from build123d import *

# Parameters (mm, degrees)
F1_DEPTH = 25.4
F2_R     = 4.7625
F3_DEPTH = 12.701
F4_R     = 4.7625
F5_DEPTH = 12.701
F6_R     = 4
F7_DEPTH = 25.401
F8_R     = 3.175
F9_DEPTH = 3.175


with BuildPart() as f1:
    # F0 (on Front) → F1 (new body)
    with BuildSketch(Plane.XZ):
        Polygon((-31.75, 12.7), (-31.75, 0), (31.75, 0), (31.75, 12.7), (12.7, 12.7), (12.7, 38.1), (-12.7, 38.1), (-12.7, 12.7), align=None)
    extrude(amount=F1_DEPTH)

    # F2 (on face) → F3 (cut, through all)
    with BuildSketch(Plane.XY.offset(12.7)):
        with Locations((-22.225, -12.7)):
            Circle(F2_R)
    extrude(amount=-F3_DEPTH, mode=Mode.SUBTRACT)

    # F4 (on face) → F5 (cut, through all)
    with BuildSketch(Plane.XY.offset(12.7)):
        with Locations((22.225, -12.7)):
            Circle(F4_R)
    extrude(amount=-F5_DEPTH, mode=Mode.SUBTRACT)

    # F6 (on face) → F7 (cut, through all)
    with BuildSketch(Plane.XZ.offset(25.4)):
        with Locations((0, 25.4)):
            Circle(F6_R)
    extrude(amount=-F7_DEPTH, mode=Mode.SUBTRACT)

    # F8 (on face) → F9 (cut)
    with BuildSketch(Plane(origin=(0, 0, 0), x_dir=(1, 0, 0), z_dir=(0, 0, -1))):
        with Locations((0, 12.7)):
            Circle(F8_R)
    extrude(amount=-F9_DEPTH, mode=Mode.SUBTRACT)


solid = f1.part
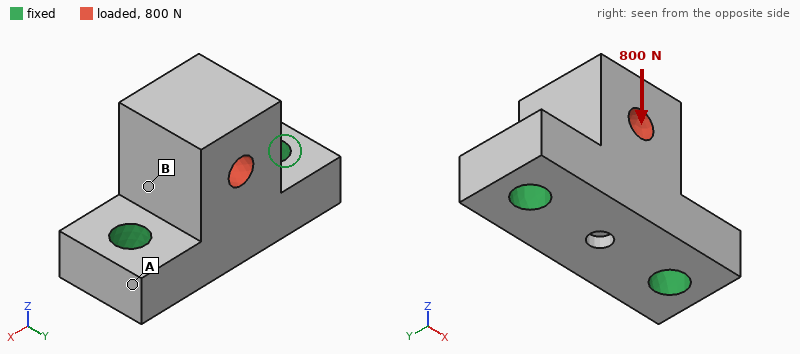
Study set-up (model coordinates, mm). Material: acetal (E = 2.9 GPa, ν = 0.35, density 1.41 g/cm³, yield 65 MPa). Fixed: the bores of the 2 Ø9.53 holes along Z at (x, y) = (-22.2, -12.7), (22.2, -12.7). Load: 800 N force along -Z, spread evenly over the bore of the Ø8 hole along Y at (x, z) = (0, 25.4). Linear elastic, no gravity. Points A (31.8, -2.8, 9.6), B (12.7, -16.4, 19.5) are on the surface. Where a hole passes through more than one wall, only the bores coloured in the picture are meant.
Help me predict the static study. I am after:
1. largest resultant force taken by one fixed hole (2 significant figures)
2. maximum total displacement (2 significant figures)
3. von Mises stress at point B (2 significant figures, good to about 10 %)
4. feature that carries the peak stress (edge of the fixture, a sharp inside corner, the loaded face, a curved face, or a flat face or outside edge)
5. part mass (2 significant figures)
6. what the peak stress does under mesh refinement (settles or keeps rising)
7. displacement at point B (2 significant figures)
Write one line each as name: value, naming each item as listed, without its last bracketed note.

largest resultant force taken by one fixed hole: 420 N
maximum total displacement: 31 µm
von Mises stress at point B: 1.3 MPa
feature that carries the peak stress: edge of the fixture
part mass: 47 g
what the peak stress does under mesh refinement: keeps rising
displacement at point B: 22 µm
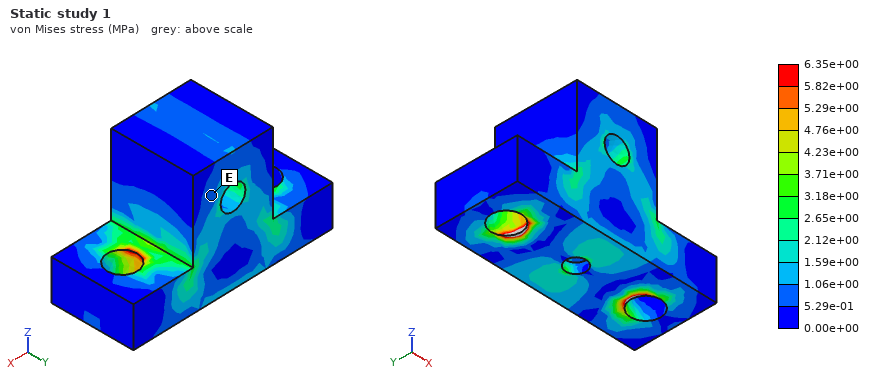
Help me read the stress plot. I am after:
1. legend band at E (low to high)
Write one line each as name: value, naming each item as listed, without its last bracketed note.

legend band at E: 5.29e-01 to 1.06e+00 MPa
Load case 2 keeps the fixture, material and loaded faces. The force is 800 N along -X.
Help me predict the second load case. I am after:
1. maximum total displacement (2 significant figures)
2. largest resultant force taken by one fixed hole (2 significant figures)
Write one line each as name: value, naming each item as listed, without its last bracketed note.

maximum total displacement: 84 µm
largest resultant force taken by one fixed hole: 580 N
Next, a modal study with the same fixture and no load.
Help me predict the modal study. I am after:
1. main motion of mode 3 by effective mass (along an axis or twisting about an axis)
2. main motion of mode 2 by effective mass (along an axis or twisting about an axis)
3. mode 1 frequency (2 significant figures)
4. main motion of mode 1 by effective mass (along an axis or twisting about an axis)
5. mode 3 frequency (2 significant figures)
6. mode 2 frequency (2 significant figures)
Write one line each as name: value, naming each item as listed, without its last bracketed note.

main motion of mode 3 by effective mass: along Z
main motion of mode 2 by effective mass: along X
mode 1 frequency: 2200 Hz
main motion of mode 1 by effective mass: along Y
mode 3 frequency: 5200 Hz
mode 2 frequency: 3800 Hz
